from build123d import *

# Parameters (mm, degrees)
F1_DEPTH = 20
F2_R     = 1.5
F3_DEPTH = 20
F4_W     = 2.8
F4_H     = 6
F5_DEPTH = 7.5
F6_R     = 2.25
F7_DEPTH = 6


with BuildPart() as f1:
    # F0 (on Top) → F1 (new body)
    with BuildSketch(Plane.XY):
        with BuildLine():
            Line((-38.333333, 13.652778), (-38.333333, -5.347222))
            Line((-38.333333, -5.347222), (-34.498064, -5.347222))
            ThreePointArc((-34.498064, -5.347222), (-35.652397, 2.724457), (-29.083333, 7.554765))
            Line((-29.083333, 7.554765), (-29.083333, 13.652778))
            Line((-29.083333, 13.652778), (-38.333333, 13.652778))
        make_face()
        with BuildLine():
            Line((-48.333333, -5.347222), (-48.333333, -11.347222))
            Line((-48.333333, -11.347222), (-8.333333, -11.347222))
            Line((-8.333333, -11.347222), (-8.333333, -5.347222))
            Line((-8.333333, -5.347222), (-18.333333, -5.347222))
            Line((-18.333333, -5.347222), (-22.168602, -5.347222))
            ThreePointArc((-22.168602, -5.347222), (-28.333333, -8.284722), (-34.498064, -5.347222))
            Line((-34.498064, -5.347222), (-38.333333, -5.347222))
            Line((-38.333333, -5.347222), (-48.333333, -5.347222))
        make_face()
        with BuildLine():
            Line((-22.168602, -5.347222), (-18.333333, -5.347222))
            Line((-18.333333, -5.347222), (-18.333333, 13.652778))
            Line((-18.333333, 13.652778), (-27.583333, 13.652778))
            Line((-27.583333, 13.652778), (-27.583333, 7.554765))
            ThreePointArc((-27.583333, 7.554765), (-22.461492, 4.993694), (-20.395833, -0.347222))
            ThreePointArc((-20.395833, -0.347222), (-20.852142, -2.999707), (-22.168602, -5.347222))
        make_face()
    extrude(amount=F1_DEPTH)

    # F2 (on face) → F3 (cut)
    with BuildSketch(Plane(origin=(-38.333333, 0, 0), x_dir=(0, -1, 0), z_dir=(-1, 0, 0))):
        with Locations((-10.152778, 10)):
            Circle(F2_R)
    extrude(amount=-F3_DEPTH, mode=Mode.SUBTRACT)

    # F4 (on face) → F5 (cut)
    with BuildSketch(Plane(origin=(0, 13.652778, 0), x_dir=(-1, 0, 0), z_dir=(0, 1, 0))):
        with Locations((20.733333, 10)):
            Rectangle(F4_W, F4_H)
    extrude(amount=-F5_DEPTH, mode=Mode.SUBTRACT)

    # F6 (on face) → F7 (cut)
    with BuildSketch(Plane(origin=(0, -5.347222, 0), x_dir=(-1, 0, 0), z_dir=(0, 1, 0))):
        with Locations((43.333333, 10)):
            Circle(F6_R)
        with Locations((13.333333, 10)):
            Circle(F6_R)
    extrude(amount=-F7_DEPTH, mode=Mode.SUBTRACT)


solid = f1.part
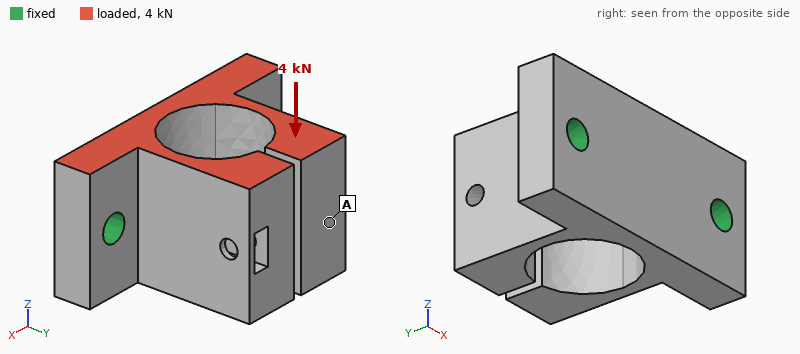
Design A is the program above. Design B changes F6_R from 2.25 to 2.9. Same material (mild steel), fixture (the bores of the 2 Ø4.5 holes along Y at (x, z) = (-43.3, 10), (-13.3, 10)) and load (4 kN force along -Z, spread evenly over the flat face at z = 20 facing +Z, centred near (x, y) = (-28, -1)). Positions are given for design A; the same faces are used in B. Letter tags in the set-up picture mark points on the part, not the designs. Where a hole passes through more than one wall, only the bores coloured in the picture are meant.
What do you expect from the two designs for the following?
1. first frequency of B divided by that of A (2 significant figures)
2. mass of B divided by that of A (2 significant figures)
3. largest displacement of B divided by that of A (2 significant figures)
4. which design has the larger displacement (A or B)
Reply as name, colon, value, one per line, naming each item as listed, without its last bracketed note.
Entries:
first frequency of B divided by that of A: 1.0
mass of B divided by that of A: 0.98
largest displacement of B divided by that of A: 0.87
which design has the larger displacement: A
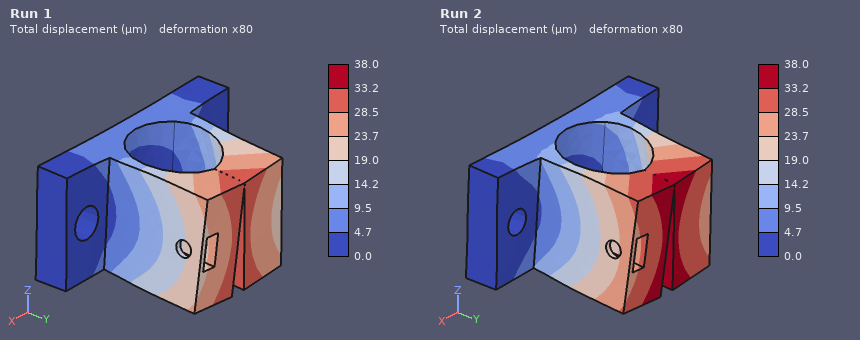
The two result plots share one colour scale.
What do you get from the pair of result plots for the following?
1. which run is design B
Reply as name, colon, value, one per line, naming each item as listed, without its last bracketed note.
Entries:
which run is design B: Run 1
